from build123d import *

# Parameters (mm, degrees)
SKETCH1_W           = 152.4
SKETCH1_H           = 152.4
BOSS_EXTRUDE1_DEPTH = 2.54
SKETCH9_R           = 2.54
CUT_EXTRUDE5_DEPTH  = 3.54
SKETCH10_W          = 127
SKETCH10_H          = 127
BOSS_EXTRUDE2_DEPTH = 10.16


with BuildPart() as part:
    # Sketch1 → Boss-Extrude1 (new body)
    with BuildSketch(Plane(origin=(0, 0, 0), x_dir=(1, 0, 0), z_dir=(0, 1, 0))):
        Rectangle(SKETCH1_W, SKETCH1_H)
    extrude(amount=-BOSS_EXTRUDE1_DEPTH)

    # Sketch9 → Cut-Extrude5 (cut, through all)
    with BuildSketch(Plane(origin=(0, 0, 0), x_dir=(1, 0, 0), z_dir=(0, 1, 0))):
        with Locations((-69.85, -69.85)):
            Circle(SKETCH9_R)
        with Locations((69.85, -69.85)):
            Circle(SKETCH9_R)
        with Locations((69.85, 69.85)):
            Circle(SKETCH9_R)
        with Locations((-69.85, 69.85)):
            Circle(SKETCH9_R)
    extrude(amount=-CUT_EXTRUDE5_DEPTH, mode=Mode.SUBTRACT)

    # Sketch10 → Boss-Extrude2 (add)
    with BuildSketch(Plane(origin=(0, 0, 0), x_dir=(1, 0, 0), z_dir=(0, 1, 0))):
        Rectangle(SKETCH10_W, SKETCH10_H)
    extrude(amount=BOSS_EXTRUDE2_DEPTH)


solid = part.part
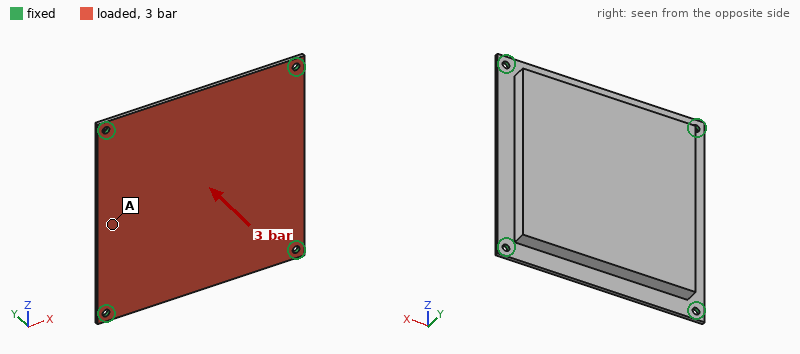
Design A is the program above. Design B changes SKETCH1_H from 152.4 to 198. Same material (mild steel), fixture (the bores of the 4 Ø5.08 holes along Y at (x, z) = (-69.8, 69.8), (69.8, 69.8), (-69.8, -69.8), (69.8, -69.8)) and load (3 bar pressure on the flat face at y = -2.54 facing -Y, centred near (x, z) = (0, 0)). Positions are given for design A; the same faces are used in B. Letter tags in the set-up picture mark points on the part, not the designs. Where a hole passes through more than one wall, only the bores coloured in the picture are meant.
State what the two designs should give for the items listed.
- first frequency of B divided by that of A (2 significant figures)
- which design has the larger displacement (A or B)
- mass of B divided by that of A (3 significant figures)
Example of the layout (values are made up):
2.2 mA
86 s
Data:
1.0
B
1.08
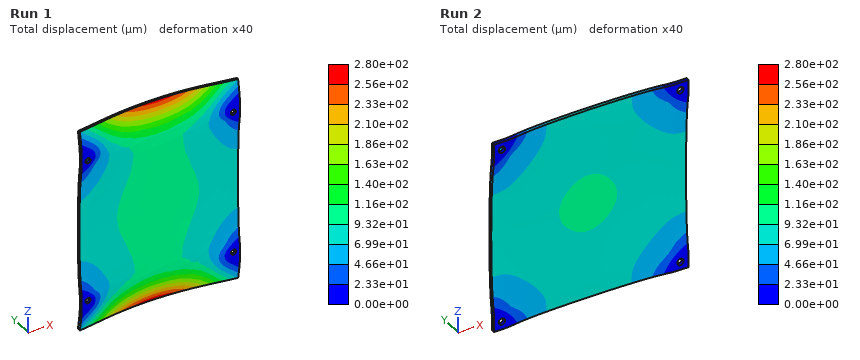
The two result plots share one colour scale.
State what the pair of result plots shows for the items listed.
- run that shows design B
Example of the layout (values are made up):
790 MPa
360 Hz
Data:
Run 1
